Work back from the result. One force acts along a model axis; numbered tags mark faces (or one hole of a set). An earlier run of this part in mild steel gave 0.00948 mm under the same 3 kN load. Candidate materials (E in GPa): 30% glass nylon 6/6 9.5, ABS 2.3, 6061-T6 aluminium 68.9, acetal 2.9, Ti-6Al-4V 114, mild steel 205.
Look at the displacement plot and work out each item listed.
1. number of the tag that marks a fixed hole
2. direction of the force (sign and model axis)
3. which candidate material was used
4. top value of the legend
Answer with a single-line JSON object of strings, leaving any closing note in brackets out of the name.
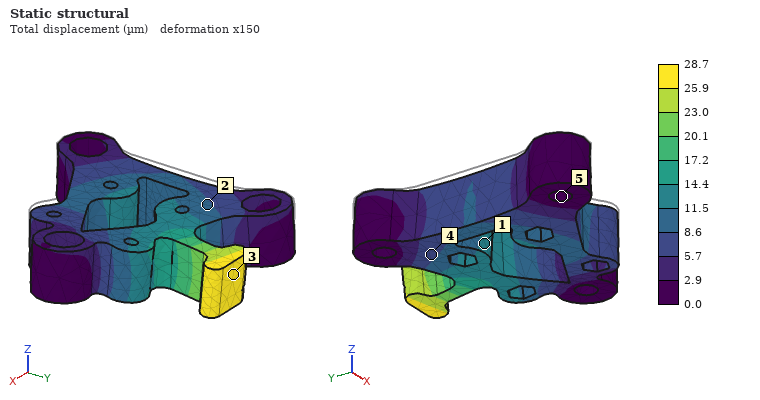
{"number of the tag that marks a fixed hole": "5", "direction of the force": "-Z", "which candidate material was used": "6061-T6 aluminium", "top value of the legend": "28.7 µm"}
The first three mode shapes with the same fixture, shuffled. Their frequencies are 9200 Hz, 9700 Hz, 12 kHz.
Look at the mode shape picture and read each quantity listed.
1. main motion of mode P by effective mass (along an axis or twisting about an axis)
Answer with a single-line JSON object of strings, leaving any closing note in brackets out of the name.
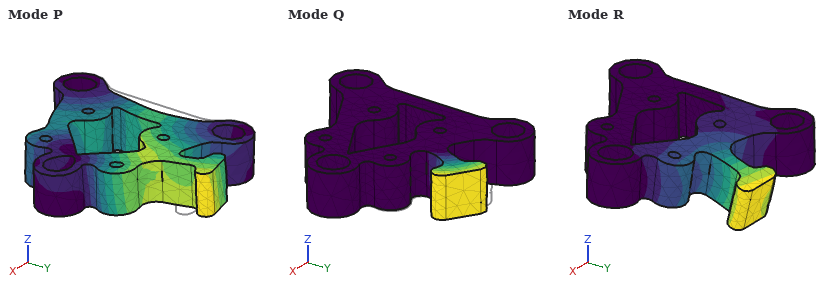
{"main motion of mode P by effective mass": "along X"}
